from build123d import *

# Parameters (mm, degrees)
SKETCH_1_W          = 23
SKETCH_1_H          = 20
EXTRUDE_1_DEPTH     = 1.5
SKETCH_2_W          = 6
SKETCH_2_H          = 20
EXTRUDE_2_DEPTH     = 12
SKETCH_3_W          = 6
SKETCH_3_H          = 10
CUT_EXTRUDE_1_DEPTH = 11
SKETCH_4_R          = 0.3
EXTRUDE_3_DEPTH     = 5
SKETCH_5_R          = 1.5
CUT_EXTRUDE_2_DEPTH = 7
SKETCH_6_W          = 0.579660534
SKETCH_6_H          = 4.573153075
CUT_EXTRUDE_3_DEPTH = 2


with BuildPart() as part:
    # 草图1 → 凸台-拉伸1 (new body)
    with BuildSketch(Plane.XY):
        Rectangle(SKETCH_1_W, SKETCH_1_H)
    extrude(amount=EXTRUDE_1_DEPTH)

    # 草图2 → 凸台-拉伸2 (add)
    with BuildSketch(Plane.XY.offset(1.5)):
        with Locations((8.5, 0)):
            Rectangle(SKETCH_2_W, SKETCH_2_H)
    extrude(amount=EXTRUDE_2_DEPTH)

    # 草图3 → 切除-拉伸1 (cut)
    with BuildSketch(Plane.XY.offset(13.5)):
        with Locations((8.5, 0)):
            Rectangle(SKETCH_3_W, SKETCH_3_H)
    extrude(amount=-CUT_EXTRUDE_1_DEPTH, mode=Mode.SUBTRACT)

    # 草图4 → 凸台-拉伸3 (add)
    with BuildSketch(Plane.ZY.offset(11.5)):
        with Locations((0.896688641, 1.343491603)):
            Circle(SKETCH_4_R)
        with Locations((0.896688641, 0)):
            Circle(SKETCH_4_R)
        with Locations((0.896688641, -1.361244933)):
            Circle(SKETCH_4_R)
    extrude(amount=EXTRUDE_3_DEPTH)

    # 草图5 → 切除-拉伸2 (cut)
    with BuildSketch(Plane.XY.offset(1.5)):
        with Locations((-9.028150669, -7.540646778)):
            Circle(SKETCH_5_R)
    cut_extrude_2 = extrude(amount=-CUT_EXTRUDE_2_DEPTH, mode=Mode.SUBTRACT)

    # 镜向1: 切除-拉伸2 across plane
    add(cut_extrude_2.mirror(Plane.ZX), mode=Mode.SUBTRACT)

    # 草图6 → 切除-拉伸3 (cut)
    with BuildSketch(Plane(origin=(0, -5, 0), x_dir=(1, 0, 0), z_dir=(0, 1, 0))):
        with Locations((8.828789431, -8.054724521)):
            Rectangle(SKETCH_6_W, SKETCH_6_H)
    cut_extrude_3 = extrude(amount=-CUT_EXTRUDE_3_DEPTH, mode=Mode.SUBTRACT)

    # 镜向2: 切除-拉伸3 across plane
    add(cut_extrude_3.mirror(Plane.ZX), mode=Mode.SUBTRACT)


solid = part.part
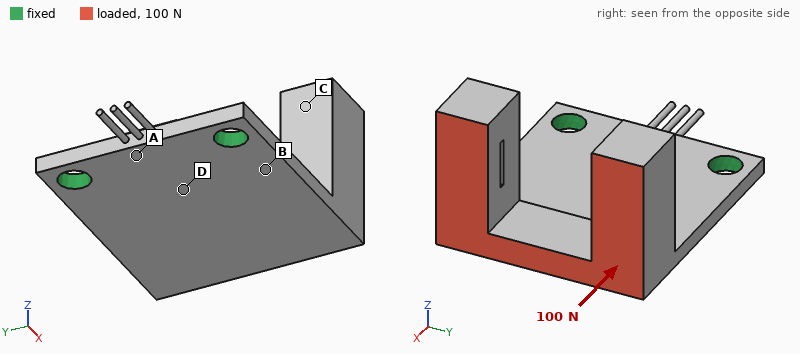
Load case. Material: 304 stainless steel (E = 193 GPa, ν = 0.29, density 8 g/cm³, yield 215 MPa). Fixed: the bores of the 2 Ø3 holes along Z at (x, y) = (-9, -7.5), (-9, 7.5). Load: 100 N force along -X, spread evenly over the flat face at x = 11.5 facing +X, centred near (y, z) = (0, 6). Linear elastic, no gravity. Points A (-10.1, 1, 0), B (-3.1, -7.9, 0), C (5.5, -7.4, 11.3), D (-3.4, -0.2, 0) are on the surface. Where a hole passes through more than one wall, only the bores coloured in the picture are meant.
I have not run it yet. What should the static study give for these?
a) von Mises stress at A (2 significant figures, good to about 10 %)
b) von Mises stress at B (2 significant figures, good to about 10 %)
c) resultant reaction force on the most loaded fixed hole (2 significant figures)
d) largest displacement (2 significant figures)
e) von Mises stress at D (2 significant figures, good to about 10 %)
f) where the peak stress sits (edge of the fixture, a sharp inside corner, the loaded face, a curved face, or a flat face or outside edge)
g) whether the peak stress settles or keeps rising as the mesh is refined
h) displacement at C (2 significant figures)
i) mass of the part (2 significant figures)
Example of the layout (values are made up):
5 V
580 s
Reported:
15 MPa
66 MPa
51 N
0.12 mm
57 MPa
edge of the fixture
keeps rising
0.087 mm
12 g
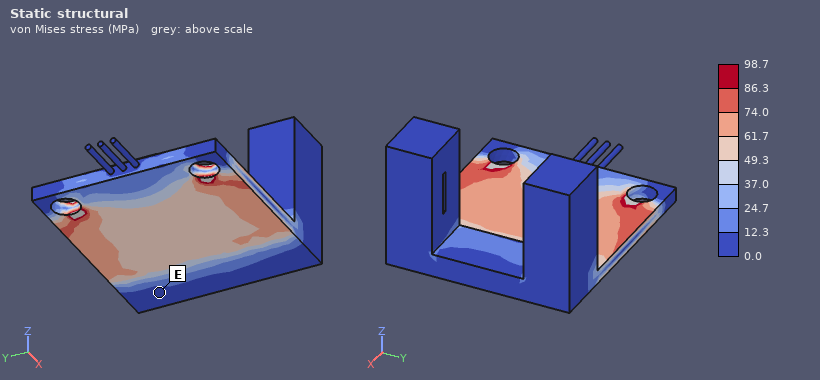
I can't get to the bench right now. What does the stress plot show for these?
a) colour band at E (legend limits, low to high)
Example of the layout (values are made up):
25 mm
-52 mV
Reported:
0.0 to 12.3 MPa
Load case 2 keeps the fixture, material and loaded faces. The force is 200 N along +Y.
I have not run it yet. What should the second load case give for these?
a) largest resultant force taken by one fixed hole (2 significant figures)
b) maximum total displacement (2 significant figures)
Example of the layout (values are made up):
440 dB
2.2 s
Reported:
280 N
81 µm
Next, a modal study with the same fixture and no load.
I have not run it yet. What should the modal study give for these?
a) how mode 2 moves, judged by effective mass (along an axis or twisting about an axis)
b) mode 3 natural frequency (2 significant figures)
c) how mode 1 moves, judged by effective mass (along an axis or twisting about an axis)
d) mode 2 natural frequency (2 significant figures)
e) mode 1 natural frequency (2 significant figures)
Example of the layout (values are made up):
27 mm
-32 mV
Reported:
along Y
5800 Hz
along Z
2700 Hz
1300 Hz
